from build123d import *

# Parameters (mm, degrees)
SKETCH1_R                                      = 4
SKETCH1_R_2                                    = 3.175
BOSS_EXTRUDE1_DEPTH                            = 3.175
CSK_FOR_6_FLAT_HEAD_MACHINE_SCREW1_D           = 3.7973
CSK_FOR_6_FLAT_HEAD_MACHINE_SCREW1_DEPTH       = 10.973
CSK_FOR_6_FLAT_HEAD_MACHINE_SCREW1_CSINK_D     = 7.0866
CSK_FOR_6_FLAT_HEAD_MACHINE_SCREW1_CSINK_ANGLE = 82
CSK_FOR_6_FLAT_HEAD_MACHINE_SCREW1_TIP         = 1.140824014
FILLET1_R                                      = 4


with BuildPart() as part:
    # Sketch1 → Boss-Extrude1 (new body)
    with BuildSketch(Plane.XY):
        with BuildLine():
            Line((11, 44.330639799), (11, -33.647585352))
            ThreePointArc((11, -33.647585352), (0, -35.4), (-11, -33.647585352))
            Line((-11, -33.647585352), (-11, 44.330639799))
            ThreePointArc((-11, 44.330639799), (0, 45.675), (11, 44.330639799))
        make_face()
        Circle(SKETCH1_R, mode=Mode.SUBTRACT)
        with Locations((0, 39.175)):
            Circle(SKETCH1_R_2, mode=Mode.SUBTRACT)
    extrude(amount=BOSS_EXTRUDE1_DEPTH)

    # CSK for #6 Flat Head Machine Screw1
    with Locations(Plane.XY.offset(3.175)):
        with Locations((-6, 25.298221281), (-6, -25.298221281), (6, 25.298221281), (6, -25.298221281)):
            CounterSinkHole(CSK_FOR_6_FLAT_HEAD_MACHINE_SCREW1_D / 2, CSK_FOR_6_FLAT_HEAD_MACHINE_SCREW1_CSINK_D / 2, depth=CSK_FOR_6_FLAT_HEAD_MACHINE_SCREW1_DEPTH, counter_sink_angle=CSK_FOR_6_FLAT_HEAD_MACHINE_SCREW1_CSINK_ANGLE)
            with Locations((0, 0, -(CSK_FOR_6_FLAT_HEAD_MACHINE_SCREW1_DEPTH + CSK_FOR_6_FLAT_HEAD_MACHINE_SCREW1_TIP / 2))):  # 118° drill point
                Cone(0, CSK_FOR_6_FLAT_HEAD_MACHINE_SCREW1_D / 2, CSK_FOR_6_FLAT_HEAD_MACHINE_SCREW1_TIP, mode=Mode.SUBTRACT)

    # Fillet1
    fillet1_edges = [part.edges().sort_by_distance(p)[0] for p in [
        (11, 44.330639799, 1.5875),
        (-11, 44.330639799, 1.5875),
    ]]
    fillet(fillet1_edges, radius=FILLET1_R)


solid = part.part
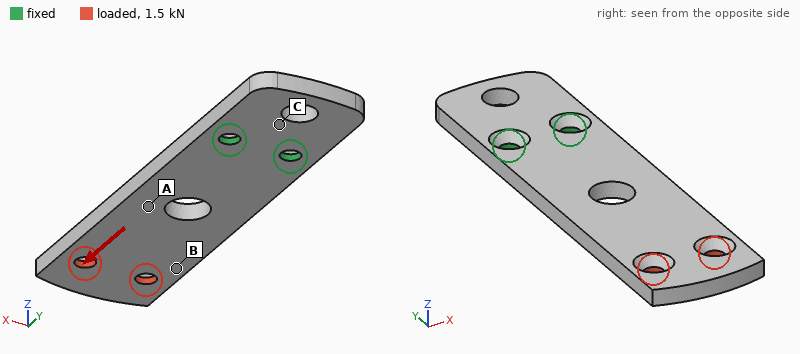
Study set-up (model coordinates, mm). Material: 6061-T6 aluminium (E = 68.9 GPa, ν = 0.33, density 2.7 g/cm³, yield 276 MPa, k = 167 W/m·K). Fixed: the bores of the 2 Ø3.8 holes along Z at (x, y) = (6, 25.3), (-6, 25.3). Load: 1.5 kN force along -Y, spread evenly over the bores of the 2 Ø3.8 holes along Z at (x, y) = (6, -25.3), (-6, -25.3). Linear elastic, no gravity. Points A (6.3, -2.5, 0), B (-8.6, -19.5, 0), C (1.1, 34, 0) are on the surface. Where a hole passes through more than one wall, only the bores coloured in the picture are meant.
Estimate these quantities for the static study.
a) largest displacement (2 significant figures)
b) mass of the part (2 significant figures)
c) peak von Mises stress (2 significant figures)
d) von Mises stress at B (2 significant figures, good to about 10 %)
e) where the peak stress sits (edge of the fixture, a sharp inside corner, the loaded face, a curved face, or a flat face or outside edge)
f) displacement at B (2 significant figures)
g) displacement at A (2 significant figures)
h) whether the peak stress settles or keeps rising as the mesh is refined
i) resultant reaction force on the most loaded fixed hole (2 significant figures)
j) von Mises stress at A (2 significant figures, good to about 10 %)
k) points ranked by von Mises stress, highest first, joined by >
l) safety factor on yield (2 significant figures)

0.66 mm
14 g
160 MPa
62 MPa
a curved face
0.36 mm
0.13 mm
settles
760 N
88 MPa
A > B > C
1.7
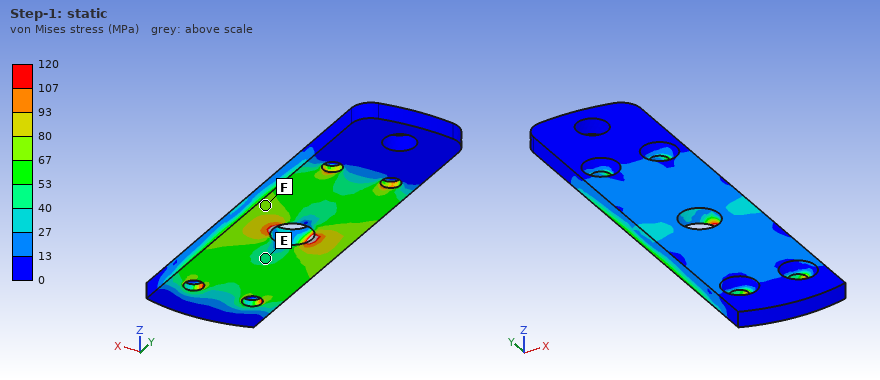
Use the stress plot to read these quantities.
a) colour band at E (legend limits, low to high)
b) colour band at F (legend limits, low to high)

40 to 53 MPa
67 to 80 MPa
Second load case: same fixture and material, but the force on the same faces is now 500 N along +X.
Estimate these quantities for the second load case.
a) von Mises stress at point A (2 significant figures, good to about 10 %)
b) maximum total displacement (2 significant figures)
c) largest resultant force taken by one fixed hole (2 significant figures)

41 MPa
0.22 mm
1.8 kN
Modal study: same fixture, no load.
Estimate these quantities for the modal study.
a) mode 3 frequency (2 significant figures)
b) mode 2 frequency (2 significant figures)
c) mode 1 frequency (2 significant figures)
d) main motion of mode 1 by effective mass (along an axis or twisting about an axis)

4000 Hz
3600 Hz
670 Hz
along Z
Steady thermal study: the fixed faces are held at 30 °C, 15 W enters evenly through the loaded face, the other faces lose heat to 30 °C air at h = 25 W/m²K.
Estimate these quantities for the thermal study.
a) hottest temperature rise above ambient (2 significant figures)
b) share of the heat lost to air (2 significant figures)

67 K
19 %
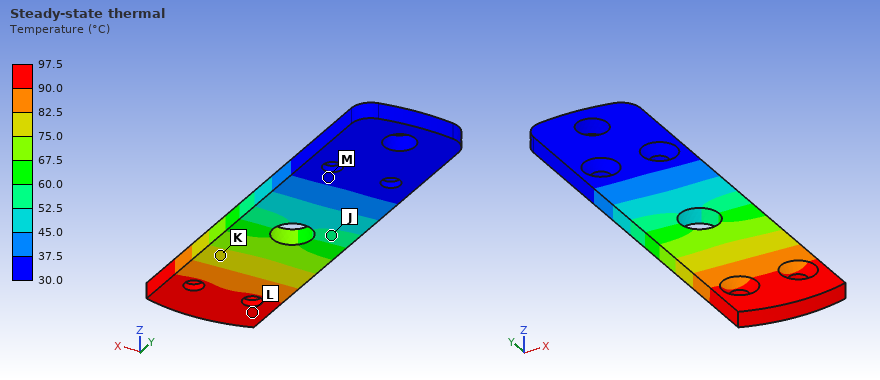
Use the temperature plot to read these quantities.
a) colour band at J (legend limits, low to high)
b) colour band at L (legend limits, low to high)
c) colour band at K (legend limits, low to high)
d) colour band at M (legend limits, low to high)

52.5 to 60.0 °C
90.0 to 97.5 °C
75.0 to 82.5 °C
30.0 to 37.5 °C
